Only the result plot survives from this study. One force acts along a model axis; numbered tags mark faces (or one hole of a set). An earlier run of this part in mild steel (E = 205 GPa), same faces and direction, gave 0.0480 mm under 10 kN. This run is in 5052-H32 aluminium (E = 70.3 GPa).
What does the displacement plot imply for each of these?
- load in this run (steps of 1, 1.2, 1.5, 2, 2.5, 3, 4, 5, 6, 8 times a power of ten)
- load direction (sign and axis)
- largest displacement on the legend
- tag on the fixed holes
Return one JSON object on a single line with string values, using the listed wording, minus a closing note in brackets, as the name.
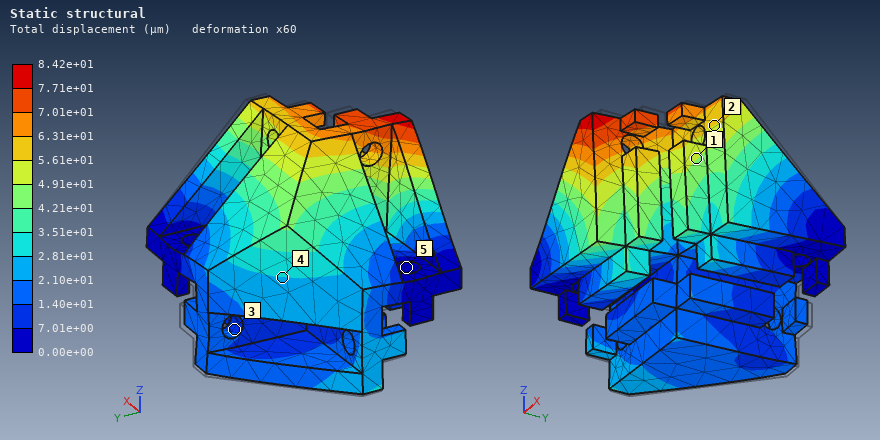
{"load in this run": "6 kN", "load direction": "-Y", "largest displacement on the legend": "8.42e+01 µm", "tag on the fixed holes": "5"}
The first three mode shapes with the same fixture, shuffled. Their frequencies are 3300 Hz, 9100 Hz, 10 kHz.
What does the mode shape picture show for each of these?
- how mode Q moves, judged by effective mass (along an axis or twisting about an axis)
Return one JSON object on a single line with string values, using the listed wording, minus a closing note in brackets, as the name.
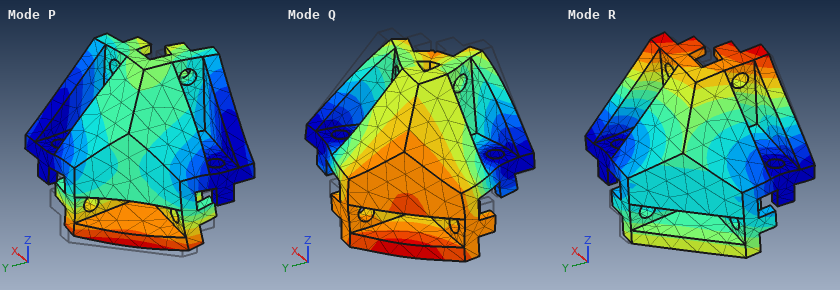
{"how mode Q moves, judged by effective mass": "along Z"}
